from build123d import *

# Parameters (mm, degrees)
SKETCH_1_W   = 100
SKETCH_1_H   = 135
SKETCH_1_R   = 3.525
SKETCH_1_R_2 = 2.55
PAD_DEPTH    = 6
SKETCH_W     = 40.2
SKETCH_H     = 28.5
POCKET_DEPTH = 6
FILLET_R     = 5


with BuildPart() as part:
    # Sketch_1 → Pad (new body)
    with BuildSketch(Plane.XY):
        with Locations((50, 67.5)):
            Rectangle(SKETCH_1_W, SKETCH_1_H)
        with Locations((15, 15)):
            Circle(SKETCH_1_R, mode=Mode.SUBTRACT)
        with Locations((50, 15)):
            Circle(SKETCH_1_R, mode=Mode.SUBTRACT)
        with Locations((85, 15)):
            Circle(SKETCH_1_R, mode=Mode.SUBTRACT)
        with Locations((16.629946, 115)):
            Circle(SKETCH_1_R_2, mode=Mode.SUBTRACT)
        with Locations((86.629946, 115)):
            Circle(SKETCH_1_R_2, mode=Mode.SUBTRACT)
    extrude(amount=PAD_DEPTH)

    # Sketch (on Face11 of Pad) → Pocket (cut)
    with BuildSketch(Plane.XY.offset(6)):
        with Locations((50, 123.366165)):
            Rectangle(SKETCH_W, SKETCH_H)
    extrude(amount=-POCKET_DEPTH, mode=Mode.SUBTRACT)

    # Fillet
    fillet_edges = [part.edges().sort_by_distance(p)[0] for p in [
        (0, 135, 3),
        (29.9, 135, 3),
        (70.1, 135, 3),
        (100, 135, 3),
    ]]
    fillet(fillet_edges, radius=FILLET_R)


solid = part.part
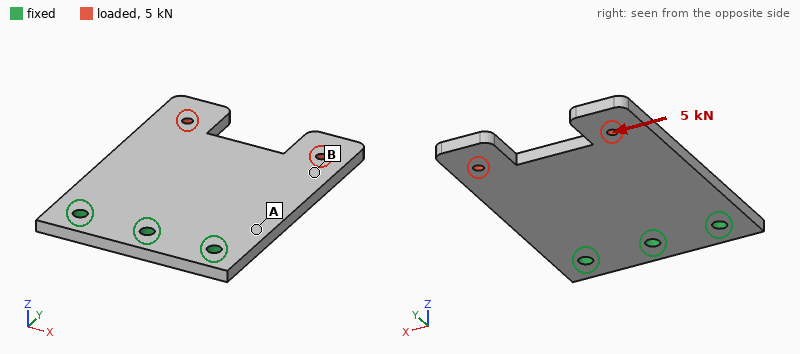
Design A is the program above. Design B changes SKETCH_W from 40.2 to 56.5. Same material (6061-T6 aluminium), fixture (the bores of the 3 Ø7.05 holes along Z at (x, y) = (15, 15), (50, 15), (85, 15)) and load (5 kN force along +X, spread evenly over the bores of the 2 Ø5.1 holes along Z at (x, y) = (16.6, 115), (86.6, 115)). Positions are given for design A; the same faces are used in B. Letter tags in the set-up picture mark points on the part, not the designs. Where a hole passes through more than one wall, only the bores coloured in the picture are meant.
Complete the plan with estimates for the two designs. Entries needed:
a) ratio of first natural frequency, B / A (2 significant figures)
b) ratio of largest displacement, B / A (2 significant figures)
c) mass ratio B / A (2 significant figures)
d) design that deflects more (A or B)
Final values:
1.1
1.2
0.97
B
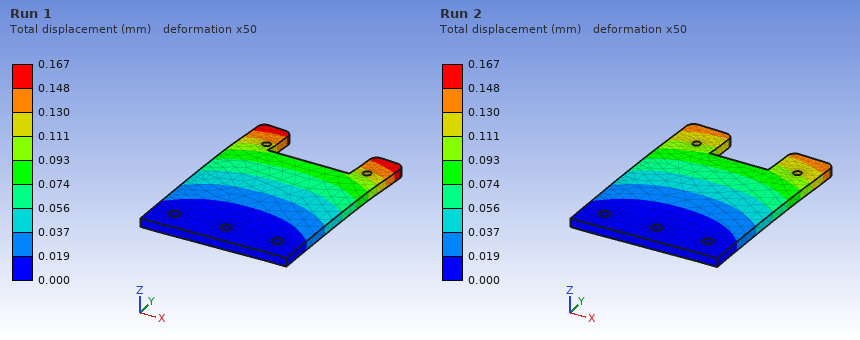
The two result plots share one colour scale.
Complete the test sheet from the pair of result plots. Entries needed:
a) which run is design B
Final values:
Run 1
